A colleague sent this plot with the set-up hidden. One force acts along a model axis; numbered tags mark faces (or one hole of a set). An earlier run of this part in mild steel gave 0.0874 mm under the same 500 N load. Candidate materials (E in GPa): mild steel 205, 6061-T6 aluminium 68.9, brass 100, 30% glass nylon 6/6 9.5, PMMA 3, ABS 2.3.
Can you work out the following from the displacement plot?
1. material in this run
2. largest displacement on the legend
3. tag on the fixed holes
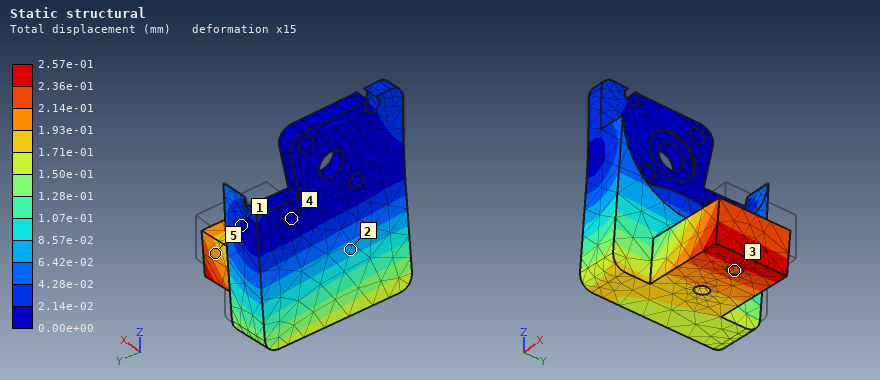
6061-T6 aluminium
2.57e-01 mm
4
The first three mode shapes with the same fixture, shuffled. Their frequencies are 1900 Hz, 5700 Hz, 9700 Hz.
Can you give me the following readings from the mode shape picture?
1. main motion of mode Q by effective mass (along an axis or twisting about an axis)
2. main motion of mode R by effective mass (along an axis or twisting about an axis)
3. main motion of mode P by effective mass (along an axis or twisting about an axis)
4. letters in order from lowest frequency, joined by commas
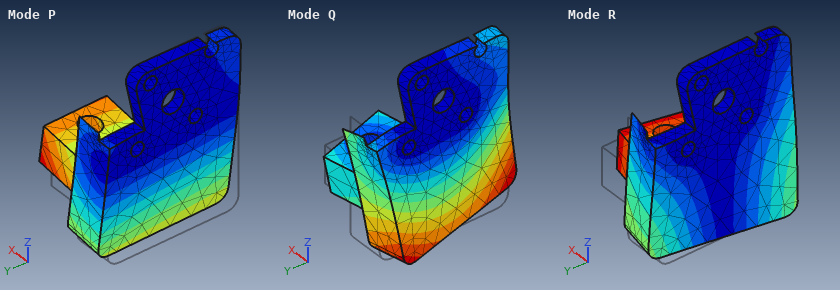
along Y
along Y
along X
P, R, Q
